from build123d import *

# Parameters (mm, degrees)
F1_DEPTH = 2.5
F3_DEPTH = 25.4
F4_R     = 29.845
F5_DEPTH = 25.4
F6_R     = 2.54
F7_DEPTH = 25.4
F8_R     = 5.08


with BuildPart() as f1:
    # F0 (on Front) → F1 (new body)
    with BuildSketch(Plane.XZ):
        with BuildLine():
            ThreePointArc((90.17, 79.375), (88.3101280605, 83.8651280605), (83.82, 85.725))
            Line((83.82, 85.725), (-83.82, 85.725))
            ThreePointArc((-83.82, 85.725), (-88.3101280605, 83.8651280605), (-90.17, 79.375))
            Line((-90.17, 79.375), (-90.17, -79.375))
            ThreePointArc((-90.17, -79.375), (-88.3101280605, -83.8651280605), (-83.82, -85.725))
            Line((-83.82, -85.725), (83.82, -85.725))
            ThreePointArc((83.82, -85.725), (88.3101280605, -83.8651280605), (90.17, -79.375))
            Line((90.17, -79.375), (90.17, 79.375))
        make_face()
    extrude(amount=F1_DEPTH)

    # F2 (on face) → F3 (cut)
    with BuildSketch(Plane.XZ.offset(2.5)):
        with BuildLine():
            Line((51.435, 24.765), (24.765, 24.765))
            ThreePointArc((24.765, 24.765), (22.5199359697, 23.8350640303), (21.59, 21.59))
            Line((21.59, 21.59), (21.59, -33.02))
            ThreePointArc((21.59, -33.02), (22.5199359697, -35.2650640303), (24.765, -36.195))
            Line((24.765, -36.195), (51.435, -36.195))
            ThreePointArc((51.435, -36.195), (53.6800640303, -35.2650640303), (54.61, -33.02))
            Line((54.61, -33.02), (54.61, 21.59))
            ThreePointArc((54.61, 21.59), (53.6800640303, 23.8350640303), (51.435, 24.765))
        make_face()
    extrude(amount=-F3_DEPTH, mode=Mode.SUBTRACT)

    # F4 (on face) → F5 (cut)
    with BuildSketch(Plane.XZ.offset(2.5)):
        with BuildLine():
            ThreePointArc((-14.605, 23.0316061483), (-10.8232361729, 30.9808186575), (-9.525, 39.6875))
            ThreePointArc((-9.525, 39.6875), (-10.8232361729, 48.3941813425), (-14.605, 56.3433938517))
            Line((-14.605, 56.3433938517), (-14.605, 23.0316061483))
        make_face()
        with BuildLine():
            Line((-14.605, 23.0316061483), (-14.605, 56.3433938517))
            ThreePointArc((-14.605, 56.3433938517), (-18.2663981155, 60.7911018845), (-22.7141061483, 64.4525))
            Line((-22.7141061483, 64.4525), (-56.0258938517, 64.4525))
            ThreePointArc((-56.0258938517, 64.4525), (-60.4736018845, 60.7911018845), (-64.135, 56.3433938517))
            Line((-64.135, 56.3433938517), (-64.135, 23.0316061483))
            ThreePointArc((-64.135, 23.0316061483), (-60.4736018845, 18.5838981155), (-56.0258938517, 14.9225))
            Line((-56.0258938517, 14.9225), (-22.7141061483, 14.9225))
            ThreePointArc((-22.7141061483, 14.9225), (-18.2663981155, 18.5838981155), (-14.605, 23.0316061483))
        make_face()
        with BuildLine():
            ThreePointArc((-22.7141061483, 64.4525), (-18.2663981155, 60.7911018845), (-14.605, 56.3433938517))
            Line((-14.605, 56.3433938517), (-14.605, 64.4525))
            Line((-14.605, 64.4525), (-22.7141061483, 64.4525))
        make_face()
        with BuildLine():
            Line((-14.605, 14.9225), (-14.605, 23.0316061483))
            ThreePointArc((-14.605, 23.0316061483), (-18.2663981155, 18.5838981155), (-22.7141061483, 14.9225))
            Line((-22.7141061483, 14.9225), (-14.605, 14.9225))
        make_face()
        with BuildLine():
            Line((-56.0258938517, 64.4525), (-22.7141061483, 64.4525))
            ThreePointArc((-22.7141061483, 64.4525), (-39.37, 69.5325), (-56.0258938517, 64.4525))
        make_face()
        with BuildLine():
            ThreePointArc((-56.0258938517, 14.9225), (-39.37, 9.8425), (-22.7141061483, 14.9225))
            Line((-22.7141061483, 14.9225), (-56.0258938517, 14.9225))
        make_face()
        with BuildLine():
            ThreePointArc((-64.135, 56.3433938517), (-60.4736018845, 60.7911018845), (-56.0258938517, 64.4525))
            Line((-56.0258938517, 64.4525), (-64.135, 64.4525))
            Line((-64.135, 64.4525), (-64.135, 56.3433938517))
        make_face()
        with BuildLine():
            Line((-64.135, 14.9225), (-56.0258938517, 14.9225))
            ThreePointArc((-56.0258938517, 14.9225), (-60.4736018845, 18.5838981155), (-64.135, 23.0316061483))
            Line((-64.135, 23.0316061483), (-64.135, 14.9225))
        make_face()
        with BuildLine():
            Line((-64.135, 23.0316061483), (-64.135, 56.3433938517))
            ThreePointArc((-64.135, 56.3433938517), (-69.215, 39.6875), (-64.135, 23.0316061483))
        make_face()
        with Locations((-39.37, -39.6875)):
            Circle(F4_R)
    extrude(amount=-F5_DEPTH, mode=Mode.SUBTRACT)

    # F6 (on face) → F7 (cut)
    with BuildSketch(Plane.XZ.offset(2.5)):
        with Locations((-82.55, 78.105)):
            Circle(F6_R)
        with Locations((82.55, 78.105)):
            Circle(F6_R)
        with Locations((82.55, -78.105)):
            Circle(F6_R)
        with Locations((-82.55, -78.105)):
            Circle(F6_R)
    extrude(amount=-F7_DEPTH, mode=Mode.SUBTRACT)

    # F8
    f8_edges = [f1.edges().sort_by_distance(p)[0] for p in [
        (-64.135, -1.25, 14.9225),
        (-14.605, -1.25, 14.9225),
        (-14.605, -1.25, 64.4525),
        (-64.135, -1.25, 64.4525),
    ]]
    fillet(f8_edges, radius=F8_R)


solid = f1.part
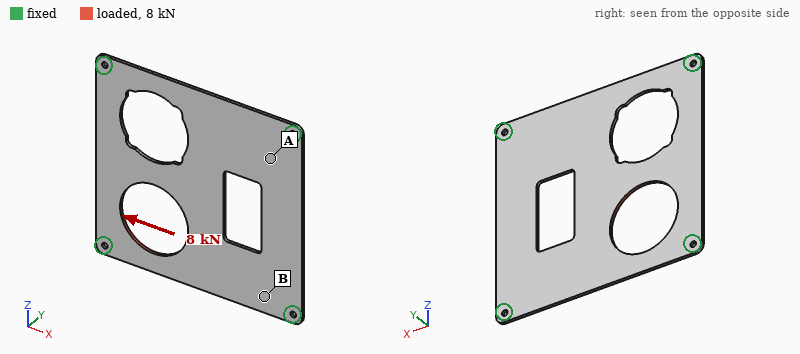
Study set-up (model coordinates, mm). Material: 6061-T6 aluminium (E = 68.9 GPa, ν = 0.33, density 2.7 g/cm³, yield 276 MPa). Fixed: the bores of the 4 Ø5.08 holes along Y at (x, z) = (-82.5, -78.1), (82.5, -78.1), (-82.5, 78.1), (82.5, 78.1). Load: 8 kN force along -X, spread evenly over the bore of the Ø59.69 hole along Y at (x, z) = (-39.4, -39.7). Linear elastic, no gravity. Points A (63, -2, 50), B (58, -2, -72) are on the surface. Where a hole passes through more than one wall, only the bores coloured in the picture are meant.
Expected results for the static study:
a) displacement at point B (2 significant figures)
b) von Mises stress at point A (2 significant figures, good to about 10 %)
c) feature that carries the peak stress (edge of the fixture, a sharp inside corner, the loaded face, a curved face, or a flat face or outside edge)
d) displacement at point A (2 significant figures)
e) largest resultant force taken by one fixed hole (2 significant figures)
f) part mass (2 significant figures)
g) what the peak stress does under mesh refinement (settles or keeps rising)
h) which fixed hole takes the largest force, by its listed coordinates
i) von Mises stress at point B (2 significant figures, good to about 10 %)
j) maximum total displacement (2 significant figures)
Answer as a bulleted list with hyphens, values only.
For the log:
- 0.019 mm
- 17 MPa
- edge of the fixture
- 0.017 mm
- 3.3 kN
- 160 g
- keeps rising
- (-82.5, -78.1)
- 35 MPa
- 0.10 mm
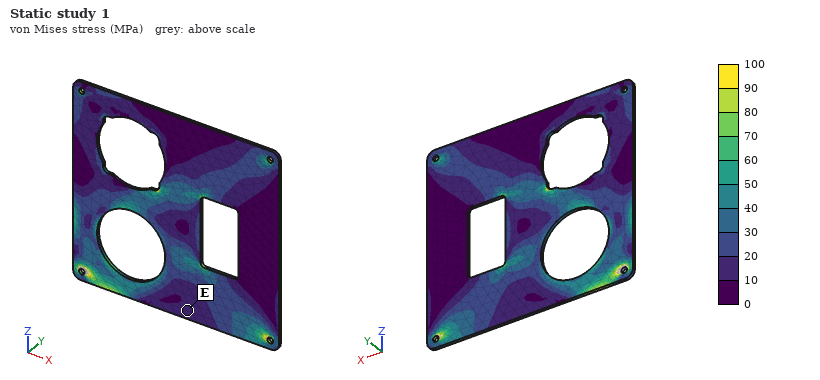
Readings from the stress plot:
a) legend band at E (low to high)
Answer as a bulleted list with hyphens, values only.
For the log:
- 10 to 20 MPa
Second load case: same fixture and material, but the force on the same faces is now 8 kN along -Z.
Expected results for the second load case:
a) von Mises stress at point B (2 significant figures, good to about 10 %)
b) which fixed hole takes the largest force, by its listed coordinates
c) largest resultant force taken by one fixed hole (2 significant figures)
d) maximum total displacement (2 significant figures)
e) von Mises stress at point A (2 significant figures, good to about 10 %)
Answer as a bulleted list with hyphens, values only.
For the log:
- 22 MPa
- (-82.5, -78.1)
- 3.2 kN
- 0.13 mm
- 14 MPa
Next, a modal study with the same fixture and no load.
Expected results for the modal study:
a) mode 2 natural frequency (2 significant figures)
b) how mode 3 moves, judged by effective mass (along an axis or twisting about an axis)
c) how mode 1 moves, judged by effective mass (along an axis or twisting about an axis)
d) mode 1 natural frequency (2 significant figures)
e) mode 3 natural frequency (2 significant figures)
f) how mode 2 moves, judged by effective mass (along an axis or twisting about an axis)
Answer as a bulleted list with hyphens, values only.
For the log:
- 510 Hz
- twisting about Z
- along Y
- 300 Hz
- 560 Hz
- twisting about X
